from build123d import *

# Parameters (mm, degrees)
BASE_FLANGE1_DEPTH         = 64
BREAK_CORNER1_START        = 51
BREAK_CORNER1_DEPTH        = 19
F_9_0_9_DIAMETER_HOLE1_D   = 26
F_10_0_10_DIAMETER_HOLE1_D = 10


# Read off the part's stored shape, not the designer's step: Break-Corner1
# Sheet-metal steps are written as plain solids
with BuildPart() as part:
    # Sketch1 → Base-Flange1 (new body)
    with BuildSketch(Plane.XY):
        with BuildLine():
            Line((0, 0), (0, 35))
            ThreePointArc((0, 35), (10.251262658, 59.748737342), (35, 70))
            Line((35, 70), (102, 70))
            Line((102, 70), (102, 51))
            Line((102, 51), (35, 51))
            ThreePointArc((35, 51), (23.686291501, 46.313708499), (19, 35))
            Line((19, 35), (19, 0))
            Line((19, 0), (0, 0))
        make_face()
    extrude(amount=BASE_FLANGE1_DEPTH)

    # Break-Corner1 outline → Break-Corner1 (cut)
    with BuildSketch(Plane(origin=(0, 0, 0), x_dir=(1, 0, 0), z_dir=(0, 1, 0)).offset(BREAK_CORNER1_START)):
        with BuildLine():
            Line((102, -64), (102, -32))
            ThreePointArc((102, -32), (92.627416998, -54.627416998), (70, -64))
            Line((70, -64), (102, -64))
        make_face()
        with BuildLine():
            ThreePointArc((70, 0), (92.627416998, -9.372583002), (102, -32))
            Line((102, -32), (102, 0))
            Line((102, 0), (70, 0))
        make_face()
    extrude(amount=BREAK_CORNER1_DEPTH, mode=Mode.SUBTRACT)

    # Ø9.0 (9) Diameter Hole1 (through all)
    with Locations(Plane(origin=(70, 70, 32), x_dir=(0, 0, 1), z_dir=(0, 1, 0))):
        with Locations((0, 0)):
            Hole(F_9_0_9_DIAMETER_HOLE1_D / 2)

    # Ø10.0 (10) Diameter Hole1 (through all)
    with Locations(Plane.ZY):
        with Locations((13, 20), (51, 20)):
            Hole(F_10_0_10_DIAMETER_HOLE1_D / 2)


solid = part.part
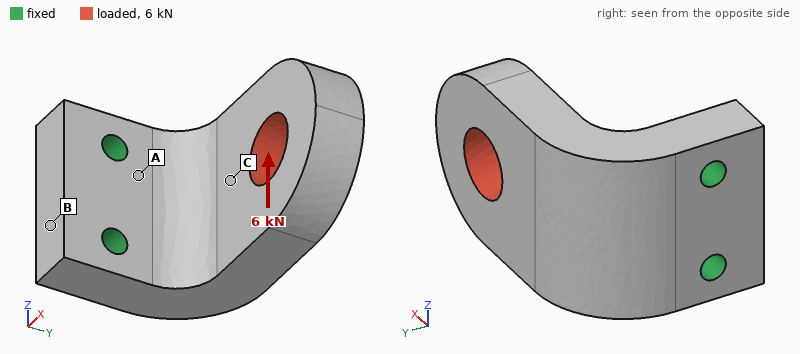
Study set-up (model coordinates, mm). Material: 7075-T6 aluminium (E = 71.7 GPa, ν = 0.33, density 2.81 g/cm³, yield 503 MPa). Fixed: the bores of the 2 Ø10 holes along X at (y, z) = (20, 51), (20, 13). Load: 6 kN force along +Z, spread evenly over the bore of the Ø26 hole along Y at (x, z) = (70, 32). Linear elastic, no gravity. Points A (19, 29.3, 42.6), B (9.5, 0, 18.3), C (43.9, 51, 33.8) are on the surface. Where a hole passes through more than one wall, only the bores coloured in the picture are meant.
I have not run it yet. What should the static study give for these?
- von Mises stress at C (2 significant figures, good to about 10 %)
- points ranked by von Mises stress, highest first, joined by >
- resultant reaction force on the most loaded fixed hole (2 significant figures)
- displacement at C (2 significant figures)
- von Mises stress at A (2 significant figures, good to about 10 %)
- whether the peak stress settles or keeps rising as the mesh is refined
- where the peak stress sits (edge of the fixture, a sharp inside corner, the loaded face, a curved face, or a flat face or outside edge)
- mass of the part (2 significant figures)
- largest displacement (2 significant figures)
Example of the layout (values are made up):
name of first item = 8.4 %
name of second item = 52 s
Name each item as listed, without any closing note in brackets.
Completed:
von Mises stress at C = 29 MPa
points ranked by von Mises stress, highest first, joined by > = A > C > B
resultant reaction force on the most loaded fixed hole = 9.5 kN
displacement at C = 0.084 mm
von Mises stress at A = 51 MPa
whether the peak stress settles or keeps rising as the mesh is refined = keeps rising
where the peak stress sits = edge of the fixture
mass of the part = 430 g
largest displacement = 0.23 mm
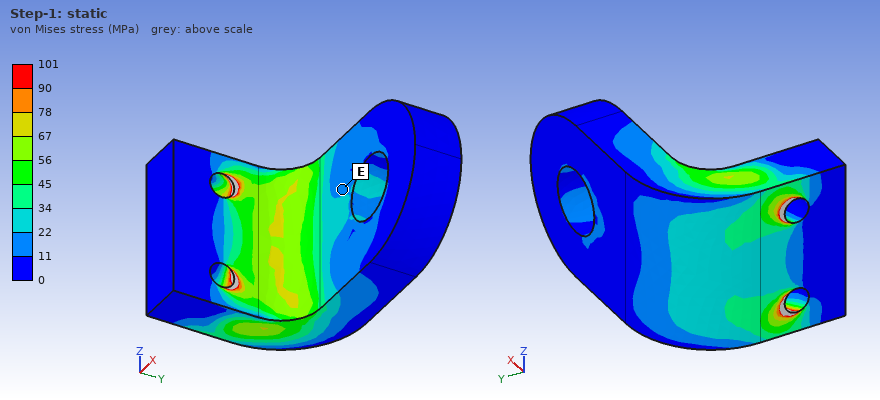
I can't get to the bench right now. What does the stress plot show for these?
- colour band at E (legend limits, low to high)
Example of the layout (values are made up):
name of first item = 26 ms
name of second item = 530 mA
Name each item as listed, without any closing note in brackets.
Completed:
colour band at E = 11 to 22 MPa
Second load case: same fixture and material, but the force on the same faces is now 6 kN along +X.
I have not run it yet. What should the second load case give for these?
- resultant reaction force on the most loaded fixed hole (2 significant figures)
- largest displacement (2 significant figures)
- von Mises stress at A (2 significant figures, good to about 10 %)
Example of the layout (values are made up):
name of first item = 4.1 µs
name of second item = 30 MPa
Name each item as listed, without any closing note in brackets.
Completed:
resultant reaction force on the most loaded fixed hole = 3.0 kN
largest displacement = 0.20 mm
von Mises stress at A = 41 MPa
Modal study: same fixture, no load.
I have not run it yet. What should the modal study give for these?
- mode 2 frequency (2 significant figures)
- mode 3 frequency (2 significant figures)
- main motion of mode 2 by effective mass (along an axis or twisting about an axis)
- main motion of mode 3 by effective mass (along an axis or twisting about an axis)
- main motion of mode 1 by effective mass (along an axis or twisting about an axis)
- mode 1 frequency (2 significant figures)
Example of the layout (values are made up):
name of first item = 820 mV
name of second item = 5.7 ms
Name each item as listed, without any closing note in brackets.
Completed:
mode 2 frequency = 2300 Hz
mode 3 frequency = 4700 Hz
main motion of mode 2 by effective mass = along Z
main motion of mode 3 by effective mass = along X
main motion of mode 1 by effective mass = along Y
mode 1 frequency = 1400 Hz
